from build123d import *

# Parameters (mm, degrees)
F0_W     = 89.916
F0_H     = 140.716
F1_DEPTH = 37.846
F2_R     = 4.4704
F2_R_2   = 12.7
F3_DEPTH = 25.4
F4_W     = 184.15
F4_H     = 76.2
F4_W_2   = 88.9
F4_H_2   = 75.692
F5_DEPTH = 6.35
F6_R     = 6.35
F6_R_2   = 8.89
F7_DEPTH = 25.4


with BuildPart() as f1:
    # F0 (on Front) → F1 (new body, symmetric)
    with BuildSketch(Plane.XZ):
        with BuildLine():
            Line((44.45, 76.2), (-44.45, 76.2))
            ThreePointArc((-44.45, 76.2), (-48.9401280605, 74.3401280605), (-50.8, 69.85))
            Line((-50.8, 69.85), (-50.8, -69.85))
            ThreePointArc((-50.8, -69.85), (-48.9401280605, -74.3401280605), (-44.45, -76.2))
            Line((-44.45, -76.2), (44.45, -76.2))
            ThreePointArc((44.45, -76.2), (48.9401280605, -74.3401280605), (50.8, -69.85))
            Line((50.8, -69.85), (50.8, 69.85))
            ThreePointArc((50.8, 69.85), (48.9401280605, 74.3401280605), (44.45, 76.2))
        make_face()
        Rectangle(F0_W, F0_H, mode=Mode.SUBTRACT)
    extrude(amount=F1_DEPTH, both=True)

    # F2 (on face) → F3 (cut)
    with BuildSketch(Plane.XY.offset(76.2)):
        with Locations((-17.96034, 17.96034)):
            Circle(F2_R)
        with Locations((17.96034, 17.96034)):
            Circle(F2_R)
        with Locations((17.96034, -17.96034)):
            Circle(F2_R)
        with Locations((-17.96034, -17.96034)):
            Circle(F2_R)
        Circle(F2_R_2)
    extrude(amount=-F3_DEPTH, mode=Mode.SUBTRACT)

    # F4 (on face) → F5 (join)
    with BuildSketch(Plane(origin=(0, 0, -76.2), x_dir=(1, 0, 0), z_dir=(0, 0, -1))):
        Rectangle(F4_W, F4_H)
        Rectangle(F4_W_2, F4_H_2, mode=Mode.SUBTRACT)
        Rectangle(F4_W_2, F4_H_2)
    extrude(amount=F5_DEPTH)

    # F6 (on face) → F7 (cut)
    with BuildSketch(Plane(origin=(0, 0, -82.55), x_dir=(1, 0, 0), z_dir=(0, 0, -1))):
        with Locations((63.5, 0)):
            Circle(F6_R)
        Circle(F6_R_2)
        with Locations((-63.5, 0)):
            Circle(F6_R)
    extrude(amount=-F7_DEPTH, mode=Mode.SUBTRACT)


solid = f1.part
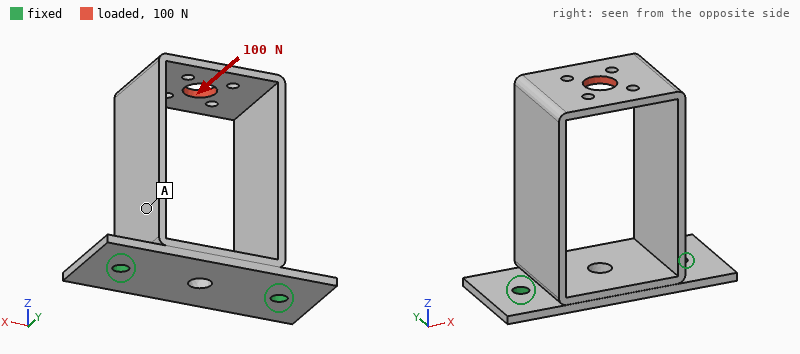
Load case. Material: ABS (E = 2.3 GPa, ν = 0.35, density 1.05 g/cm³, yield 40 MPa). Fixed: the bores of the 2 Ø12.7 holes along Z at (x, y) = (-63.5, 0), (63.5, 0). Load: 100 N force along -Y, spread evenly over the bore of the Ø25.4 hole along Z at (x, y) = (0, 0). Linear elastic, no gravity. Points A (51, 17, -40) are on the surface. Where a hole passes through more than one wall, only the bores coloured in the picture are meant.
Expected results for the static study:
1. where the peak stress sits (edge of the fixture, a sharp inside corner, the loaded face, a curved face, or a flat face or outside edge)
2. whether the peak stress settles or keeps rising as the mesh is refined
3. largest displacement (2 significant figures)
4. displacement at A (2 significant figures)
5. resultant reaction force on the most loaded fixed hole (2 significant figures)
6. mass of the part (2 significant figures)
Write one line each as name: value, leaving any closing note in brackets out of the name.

where the peak stress sits: edge of the fixture
whether the peak stress settles or keeps rising as the mesh is refined: keeps rising
largest displacement: 2.9 mm
displacement at A: 0.76 mm
resultant reaction force on the most loaded fixed hole: 50 N
mass of the part: 310 g
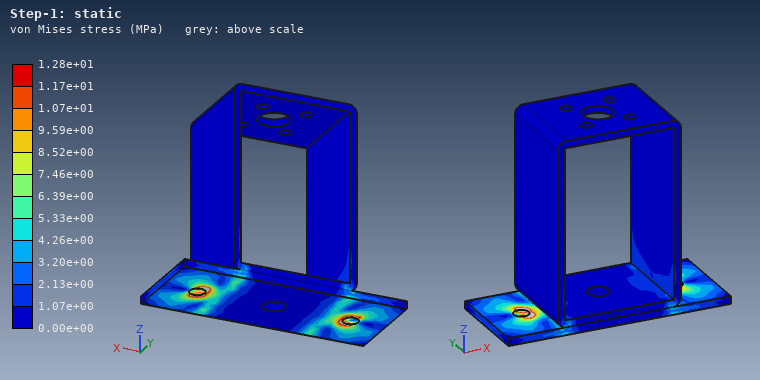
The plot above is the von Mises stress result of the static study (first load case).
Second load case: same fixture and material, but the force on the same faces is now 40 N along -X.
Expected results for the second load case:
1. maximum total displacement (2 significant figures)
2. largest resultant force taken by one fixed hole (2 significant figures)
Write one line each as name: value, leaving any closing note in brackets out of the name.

maximum total displacement: 2.5 mm
largest resultant force taken by one fixed hole: 60 N
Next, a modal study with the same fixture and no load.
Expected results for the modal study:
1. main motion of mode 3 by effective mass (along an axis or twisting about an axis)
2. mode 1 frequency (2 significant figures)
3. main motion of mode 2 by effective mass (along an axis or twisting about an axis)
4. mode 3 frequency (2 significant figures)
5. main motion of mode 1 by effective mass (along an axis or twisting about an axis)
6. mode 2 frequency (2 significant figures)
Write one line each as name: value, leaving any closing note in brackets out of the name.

main motion of mode 3 by effective mass: twisting about Z
mode 1 frequency: 69 Hz
main motion of mode 2 by effective mass: along Y
mode 3 frequency: 220 Hz
main motion of mode 1 by effective mass: along X
mode 2 frequency: 100 Hz
